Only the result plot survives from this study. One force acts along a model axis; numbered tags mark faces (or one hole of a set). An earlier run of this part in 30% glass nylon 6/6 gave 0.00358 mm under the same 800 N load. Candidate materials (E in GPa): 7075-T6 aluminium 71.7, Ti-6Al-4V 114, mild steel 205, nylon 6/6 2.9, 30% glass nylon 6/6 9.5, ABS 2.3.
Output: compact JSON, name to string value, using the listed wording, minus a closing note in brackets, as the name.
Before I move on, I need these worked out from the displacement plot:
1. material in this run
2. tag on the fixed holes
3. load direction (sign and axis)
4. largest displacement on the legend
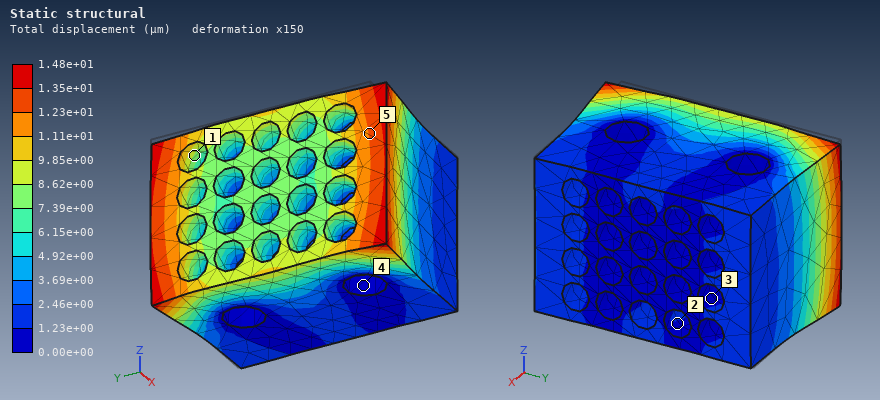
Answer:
{"material in this run": "ABS", "tag on the fixed holes": "4", "load direction": "+X", "largest displacement on the legend": "1.48e+01 µm"}
